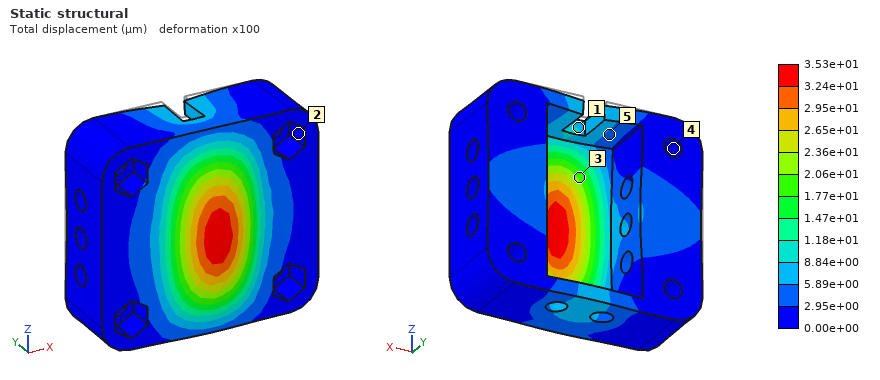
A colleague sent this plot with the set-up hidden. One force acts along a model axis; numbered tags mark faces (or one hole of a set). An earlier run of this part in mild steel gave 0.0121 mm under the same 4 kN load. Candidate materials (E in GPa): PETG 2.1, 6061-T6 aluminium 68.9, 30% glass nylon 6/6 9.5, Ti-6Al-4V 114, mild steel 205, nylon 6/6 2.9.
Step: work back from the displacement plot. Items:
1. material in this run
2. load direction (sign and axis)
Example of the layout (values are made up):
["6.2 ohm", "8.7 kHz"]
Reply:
["6061-T6 aluminium", "-Y"]
